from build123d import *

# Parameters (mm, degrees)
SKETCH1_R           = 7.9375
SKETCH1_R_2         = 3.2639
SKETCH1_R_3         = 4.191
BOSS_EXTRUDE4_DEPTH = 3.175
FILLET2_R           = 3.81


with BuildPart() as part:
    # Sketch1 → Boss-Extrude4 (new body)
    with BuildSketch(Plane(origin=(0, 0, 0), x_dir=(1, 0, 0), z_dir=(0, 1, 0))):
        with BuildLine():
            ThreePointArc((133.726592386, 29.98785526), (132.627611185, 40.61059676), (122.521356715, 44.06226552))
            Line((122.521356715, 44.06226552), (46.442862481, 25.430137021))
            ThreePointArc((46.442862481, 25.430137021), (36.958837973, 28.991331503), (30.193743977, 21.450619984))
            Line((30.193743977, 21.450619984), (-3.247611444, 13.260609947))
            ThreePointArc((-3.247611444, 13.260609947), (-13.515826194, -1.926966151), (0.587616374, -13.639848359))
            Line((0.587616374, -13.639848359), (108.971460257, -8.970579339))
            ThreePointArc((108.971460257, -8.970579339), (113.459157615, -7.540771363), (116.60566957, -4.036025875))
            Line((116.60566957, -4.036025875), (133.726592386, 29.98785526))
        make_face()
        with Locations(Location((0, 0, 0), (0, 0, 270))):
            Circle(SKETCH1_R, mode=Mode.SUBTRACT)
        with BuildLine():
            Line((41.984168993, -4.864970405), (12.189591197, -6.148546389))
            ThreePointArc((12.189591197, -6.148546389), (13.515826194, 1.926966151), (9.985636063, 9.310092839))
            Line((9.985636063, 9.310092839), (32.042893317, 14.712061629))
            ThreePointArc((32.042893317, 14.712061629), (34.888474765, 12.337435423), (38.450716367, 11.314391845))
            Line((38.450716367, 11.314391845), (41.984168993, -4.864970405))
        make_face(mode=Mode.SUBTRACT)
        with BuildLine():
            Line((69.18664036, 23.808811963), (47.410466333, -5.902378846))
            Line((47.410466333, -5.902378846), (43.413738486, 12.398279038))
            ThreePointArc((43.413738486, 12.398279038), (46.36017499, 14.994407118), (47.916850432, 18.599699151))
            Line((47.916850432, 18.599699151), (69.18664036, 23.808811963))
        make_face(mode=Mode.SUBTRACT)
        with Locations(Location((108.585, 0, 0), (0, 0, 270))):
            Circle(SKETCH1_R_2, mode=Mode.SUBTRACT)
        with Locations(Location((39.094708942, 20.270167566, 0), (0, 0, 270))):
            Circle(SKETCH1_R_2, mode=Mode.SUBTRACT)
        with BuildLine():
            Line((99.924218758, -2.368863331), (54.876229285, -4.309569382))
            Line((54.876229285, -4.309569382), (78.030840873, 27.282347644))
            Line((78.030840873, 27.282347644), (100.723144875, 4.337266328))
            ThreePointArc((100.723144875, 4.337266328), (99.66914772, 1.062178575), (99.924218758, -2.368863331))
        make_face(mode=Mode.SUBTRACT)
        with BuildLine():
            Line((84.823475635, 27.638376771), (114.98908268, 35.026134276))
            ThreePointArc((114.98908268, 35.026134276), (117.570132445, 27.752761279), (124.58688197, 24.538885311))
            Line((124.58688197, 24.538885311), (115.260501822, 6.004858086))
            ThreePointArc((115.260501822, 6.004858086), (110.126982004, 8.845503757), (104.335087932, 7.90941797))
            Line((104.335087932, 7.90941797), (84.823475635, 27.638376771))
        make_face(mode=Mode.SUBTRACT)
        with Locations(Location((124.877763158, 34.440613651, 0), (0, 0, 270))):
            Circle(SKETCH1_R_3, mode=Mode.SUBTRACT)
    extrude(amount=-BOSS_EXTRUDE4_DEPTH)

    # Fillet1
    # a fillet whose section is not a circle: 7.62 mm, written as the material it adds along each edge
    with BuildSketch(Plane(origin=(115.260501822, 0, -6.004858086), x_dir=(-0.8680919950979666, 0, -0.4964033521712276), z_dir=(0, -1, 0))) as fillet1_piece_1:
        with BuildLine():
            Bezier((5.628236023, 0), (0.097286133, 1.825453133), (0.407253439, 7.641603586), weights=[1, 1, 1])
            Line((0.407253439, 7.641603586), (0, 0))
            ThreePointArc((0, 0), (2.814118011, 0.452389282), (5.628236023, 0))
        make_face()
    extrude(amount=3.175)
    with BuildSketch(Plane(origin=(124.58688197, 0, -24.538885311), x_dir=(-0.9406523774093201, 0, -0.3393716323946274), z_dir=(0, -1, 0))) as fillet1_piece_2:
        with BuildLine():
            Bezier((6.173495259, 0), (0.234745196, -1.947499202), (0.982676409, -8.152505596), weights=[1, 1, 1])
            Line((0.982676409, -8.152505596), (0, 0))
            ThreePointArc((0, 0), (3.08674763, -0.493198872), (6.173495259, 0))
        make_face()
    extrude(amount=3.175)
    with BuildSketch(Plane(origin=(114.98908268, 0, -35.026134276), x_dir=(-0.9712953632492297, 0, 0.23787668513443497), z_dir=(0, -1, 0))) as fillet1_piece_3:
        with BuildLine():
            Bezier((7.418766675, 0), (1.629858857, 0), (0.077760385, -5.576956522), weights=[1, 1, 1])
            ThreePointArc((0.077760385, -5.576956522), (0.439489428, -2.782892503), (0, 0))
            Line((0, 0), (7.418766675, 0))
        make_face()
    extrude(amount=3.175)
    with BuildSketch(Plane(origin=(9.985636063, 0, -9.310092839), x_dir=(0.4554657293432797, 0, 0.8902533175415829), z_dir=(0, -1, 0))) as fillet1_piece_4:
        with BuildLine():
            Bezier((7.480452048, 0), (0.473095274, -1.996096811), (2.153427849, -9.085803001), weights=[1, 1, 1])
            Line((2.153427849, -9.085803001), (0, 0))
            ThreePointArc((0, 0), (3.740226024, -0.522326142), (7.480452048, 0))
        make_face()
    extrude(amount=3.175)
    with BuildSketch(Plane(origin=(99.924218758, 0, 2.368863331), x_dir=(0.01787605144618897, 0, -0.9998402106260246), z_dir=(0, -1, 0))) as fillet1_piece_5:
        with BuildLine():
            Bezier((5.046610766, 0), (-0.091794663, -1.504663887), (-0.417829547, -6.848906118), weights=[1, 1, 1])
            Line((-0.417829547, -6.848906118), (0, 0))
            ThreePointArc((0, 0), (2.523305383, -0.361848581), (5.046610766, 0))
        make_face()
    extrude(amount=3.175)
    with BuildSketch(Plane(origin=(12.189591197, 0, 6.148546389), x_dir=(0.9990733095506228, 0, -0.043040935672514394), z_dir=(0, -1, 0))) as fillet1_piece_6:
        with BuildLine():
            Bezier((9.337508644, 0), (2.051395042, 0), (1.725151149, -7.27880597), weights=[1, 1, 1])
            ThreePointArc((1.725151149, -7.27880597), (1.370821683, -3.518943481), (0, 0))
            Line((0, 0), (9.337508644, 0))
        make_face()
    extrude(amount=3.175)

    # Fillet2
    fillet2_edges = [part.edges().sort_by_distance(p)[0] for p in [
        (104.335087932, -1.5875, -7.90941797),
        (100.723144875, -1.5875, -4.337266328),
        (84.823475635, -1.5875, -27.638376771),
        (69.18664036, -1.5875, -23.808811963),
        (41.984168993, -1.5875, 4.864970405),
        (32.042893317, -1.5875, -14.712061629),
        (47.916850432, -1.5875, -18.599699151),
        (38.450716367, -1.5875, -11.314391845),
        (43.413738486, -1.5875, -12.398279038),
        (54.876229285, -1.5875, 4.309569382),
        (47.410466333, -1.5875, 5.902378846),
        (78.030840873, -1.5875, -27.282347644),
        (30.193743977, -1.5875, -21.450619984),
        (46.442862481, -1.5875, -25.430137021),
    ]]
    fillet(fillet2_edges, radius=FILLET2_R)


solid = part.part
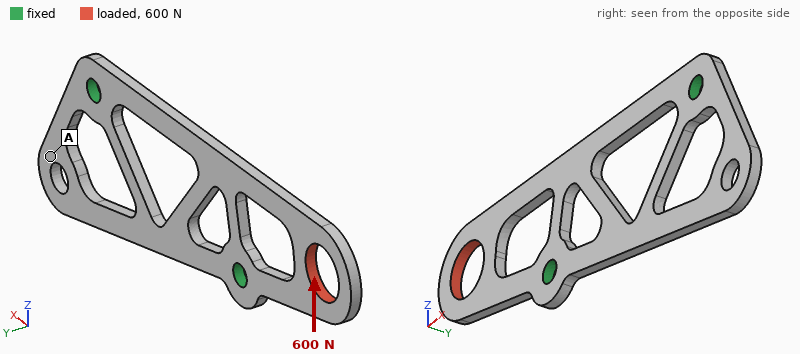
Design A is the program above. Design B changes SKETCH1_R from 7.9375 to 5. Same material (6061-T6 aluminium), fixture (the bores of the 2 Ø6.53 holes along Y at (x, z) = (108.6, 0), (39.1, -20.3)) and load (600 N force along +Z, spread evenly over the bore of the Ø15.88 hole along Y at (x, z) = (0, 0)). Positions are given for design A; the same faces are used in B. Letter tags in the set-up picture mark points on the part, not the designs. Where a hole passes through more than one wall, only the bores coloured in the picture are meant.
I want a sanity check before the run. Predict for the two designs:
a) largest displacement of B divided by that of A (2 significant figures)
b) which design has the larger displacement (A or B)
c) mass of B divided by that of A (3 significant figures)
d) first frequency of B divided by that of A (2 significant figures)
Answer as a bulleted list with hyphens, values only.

- 0.85
- A
- 1.04
- 0.90
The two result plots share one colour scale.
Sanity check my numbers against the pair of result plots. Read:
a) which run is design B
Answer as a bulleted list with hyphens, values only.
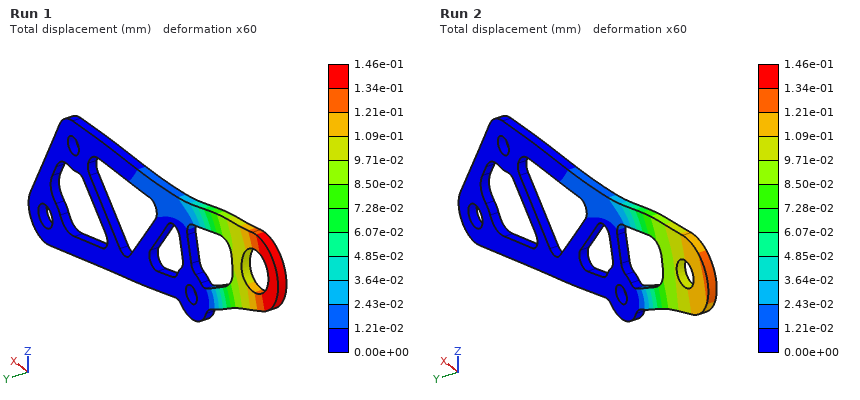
- Run 2
